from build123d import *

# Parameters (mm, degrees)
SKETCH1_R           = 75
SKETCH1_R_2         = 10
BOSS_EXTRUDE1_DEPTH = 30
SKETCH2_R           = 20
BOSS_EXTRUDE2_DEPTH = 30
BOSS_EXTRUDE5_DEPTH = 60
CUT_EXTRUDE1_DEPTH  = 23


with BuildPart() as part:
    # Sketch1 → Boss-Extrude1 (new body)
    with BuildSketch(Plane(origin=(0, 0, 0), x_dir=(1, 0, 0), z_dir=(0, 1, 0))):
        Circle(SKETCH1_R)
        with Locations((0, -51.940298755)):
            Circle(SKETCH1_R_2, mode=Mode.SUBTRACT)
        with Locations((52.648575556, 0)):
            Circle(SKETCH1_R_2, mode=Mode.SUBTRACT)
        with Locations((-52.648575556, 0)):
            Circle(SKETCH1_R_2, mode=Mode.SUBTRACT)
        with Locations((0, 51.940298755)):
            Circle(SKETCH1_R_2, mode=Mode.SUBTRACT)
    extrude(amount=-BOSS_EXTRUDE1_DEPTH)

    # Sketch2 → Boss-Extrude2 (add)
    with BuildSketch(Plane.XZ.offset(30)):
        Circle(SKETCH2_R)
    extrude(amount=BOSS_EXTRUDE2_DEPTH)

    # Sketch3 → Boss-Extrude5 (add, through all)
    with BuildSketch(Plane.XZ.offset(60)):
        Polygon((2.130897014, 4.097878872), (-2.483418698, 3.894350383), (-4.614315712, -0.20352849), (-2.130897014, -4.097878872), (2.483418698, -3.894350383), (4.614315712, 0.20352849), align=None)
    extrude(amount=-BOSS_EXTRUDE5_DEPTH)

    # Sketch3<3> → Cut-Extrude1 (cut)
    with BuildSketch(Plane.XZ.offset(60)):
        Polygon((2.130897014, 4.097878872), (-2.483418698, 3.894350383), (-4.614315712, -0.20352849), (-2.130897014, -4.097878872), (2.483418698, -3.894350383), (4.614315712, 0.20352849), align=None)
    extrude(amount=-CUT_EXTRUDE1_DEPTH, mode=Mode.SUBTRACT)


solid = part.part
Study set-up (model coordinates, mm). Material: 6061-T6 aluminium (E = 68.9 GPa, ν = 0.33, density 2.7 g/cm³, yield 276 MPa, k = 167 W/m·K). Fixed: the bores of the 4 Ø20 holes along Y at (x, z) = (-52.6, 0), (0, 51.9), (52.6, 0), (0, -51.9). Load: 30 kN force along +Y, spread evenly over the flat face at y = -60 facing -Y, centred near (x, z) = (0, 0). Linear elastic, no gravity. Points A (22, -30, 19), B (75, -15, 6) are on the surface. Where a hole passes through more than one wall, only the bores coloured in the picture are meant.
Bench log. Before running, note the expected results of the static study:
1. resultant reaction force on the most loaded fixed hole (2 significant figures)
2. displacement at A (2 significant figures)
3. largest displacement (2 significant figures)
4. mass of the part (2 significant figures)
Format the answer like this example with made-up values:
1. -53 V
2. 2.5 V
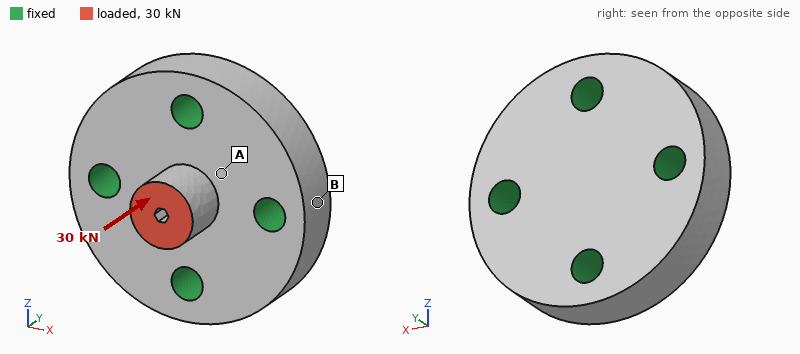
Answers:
1. 7.9 kN
2. 7.0 µm
3. 24 µm
4. 1.4 kg
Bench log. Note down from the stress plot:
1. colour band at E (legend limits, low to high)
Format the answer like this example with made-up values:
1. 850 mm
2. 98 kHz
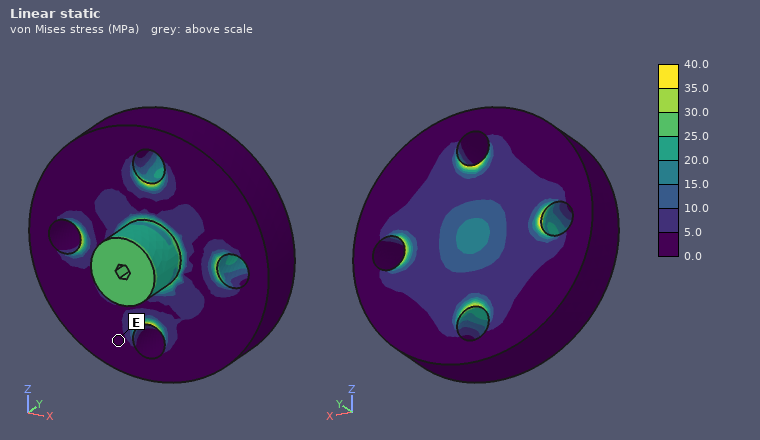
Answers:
1. 0.0 to 5.0 MPa
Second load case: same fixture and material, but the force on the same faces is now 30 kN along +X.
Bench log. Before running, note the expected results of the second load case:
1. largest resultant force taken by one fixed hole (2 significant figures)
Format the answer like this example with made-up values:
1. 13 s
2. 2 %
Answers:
1. 18 kN
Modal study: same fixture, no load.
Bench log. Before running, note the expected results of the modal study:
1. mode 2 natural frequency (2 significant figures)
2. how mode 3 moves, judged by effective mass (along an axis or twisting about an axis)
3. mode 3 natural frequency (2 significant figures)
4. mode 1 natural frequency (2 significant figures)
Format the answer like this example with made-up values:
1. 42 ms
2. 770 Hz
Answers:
1. 12 kHz
2. along Y
3. 14 kHz
4. 12 kHz
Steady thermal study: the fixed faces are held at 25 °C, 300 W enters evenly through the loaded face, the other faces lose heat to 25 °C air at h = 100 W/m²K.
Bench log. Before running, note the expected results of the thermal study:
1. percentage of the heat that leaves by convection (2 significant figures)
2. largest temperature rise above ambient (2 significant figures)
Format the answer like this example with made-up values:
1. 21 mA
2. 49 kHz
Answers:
1. 9.0 %
2. 62 K
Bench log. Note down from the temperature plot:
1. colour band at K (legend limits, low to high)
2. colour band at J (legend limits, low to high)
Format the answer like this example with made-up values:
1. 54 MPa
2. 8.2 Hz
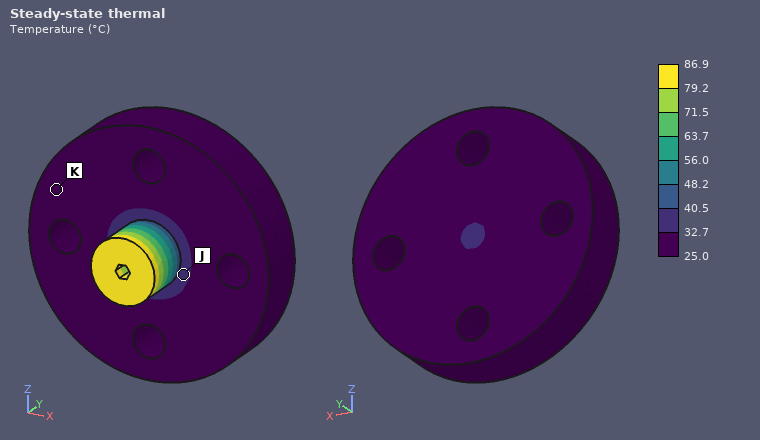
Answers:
1. 25.0 to 32.7 °C
2. 32.7 to 40.5 °C
